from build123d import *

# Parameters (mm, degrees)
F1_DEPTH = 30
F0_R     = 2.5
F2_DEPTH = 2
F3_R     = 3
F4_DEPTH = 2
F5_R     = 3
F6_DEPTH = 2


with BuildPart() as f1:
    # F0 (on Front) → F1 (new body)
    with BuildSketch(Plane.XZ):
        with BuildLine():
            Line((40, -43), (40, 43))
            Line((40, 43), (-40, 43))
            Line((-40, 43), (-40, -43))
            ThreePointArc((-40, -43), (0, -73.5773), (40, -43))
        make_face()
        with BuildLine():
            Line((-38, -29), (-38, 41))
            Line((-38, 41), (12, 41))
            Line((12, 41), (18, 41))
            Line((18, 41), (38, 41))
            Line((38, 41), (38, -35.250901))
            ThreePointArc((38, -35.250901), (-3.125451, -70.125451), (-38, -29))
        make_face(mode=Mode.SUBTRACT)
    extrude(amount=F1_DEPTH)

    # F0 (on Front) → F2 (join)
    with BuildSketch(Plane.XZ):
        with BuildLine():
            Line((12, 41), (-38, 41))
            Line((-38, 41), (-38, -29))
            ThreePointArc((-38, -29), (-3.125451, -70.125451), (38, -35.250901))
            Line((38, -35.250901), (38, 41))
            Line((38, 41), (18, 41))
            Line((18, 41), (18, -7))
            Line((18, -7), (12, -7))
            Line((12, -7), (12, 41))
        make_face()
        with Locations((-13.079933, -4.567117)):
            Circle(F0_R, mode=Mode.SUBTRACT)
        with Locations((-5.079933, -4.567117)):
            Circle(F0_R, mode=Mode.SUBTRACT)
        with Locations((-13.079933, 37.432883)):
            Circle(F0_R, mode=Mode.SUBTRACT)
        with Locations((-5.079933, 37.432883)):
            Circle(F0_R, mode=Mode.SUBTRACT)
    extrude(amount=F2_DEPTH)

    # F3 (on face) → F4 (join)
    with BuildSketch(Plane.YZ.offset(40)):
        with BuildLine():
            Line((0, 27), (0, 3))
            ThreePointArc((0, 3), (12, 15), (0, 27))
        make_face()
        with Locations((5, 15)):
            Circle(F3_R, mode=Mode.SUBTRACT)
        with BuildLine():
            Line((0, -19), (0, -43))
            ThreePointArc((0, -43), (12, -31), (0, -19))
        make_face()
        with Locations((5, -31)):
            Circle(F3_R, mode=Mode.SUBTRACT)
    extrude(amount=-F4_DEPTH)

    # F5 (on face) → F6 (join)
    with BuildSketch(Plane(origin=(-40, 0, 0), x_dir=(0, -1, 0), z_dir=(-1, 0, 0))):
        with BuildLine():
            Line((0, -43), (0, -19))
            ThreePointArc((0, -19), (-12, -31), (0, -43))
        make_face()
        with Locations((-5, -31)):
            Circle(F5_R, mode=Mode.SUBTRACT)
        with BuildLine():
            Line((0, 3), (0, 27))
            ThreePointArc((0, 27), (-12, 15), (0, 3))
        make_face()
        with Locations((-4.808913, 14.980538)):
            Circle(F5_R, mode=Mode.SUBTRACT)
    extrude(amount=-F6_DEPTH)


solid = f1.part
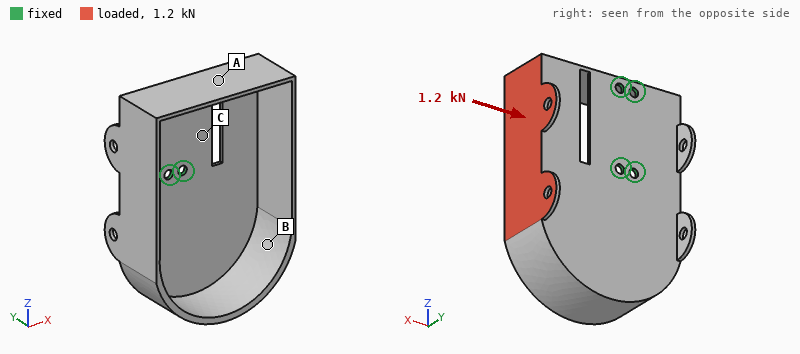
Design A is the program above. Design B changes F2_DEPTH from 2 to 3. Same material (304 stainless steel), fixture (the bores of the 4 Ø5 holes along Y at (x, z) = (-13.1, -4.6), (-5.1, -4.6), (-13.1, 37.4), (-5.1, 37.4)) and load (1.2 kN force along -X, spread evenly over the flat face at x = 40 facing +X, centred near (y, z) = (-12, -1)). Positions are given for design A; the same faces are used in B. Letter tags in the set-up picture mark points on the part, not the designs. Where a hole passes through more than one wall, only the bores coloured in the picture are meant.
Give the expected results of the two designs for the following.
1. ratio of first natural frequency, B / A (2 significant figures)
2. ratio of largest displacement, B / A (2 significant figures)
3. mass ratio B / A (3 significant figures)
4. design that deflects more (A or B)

1.4
0.59
1.18
A
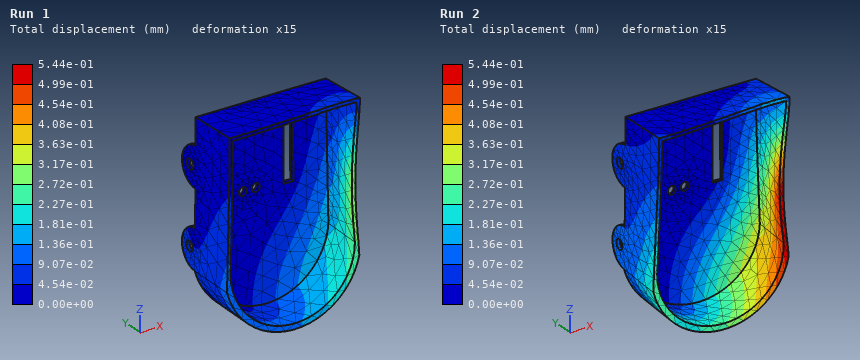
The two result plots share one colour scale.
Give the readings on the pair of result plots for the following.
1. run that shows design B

Run 1
